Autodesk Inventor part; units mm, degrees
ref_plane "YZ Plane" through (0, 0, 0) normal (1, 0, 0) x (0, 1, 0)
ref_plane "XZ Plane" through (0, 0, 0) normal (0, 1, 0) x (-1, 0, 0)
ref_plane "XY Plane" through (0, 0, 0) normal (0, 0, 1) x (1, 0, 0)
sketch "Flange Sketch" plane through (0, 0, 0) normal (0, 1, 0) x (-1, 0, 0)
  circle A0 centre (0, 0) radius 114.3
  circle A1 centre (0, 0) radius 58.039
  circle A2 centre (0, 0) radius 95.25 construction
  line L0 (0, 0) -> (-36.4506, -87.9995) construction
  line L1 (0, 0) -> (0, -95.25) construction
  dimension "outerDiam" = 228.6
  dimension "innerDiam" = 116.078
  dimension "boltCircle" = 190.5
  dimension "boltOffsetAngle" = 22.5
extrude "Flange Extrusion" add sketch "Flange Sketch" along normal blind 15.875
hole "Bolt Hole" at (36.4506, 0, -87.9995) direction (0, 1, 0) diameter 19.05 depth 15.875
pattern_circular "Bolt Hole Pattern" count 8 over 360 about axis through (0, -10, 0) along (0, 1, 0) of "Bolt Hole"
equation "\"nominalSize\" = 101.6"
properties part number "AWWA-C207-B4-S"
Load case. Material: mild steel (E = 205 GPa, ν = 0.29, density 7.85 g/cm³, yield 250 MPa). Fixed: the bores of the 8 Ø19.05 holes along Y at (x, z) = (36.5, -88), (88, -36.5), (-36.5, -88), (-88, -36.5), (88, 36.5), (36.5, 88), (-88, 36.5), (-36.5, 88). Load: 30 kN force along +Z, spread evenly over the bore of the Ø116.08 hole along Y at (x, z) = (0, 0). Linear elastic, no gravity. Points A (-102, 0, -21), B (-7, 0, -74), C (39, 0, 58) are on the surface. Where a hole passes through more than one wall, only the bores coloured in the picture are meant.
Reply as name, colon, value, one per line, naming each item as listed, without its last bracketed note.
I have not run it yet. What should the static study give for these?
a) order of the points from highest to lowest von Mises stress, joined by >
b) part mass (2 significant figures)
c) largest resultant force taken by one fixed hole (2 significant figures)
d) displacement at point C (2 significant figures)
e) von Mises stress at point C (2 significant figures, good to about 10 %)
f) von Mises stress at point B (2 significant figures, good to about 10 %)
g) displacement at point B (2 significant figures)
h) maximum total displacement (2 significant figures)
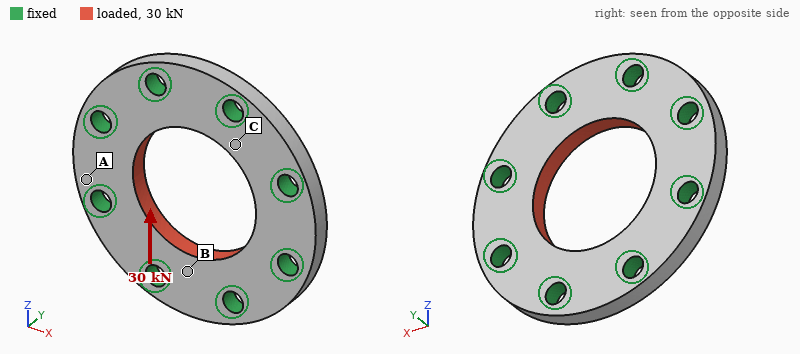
order of the points from highest to lowest von Mises stress, joined by >: C > B > A
part mass: 3.5 kg
largest resultant force taken by one fixed hole: 4.9 kN
displacement at point C: 0.76 µm
von Mises stress at point C: 6.9 MPa
von Mises stress at point B: 3.6 MPa
displacement at point B: 0.91 µm
maximum total displacement: 1.4 µm
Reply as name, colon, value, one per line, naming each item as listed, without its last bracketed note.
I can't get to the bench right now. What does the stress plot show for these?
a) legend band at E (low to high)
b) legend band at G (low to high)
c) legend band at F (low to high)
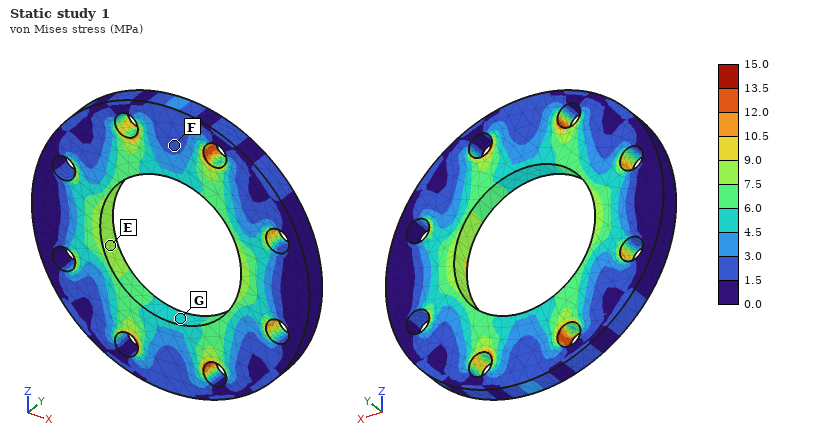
legend band at E: 7.5 to 9.0 MPa
legend band at G: 4.5 to 6.0 MPa
legend band at F: 1.5 to 3.0 MPa
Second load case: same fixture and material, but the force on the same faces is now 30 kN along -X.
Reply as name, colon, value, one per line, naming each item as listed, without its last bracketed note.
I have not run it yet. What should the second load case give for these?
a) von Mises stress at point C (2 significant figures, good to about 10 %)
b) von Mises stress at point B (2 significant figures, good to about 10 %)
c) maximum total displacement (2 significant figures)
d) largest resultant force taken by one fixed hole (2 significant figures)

von Mises stress at point C: 4.1 MPa
von Mises stress at point B: 5.3 MPa
maximum total displacement: 1.4 µm
largest resultant force taken by one fixed hole: 4.9 kN
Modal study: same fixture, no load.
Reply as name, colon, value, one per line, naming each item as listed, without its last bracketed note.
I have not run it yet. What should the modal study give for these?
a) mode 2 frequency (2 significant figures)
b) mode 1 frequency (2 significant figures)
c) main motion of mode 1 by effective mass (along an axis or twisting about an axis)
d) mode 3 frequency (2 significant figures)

mode 2 frequency: 11 kHz
mode 1 frequency: 10 kHz
main motion of mode 1 by effective mass: along Y
mode 3 frequency: 11 kHz
